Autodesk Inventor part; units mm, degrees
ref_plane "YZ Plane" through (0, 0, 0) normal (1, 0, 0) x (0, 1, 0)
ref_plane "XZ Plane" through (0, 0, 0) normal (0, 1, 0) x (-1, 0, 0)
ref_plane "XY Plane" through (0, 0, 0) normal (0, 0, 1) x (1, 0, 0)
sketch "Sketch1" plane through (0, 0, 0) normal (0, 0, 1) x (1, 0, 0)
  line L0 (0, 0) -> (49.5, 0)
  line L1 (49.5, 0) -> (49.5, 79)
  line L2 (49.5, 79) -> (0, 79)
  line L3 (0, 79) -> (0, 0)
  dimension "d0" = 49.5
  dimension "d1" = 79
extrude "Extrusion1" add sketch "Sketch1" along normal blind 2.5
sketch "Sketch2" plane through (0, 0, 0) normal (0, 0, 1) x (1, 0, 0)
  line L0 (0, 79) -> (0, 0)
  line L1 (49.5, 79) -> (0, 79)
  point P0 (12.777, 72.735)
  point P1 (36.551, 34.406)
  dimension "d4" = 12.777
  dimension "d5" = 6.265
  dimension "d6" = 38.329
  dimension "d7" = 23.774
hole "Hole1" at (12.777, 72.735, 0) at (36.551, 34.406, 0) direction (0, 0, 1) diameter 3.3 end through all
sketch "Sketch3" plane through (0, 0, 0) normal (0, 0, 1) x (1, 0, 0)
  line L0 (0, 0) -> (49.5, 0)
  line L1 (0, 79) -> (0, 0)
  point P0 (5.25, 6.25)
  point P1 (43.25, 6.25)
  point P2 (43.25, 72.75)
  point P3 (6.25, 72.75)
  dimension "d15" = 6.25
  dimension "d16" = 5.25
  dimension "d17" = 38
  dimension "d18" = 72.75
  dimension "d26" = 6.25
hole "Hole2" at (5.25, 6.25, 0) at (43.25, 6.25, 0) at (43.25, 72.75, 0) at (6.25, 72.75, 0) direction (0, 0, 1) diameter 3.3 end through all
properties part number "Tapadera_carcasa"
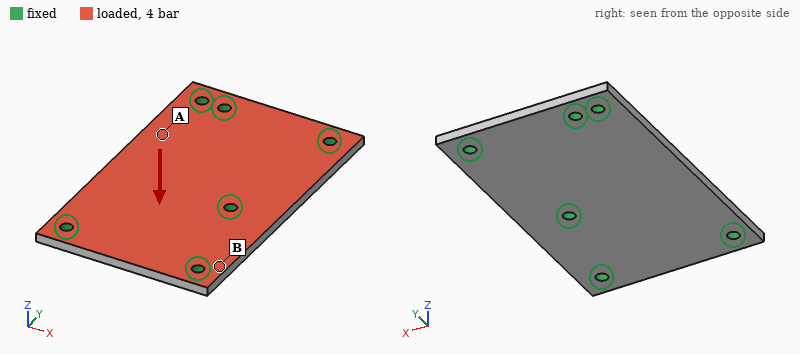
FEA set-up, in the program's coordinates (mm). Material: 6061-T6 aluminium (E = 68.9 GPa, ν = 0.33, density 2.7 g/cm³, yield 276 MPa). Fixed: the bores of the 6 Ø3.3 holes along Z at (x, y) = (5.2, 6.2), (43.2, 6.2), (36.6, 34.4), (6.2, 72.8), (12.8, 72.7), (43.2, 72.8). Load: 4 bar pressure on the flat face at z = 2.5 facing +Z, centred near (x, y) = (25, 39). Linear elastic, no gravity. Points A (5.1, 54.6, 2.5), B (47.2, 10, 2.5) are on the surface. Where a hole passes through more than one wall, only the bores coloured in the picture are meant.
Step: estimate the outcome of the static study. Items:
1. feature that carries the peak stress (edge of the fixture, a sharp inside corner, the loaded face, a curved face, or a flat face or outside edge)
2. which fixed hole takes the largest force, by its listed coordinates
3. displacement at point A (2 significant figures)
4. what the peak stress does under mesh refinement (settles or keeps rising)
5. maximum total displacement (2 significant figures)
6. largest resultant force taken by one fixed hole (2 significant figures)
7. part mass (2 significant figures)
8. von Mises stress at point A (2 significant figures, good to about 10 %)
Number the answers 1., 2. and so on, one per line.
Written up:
1. edge of the fixture
2. (36.6, 34.4)
3. 0.10 mm
4. keeps rising
5. 0.18 mm
6. 520 N
7. 26 g
8. 32 MPa
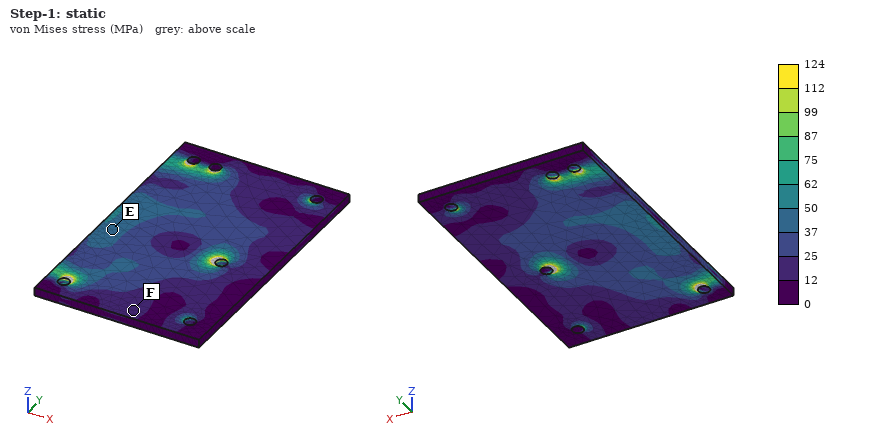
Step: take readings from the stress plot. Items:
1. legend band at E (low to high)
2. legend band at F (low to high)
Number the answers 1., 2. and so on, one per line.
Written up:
1. 37 to 50 MPa
2. 12 to 25 MPa
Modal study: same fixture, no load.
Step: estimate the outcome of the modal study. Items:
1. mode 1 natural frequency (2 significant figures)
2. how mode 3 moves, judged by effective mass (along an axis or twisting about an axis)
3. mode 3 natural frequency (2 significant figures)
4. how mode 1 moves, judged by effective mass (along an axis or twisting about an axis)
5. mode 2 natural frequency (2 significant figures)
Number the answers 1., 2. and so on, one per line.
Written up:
1. 3800 Hz
2. along Z
3. 8500 Hz
4. along Z
5. 7700 Hz
